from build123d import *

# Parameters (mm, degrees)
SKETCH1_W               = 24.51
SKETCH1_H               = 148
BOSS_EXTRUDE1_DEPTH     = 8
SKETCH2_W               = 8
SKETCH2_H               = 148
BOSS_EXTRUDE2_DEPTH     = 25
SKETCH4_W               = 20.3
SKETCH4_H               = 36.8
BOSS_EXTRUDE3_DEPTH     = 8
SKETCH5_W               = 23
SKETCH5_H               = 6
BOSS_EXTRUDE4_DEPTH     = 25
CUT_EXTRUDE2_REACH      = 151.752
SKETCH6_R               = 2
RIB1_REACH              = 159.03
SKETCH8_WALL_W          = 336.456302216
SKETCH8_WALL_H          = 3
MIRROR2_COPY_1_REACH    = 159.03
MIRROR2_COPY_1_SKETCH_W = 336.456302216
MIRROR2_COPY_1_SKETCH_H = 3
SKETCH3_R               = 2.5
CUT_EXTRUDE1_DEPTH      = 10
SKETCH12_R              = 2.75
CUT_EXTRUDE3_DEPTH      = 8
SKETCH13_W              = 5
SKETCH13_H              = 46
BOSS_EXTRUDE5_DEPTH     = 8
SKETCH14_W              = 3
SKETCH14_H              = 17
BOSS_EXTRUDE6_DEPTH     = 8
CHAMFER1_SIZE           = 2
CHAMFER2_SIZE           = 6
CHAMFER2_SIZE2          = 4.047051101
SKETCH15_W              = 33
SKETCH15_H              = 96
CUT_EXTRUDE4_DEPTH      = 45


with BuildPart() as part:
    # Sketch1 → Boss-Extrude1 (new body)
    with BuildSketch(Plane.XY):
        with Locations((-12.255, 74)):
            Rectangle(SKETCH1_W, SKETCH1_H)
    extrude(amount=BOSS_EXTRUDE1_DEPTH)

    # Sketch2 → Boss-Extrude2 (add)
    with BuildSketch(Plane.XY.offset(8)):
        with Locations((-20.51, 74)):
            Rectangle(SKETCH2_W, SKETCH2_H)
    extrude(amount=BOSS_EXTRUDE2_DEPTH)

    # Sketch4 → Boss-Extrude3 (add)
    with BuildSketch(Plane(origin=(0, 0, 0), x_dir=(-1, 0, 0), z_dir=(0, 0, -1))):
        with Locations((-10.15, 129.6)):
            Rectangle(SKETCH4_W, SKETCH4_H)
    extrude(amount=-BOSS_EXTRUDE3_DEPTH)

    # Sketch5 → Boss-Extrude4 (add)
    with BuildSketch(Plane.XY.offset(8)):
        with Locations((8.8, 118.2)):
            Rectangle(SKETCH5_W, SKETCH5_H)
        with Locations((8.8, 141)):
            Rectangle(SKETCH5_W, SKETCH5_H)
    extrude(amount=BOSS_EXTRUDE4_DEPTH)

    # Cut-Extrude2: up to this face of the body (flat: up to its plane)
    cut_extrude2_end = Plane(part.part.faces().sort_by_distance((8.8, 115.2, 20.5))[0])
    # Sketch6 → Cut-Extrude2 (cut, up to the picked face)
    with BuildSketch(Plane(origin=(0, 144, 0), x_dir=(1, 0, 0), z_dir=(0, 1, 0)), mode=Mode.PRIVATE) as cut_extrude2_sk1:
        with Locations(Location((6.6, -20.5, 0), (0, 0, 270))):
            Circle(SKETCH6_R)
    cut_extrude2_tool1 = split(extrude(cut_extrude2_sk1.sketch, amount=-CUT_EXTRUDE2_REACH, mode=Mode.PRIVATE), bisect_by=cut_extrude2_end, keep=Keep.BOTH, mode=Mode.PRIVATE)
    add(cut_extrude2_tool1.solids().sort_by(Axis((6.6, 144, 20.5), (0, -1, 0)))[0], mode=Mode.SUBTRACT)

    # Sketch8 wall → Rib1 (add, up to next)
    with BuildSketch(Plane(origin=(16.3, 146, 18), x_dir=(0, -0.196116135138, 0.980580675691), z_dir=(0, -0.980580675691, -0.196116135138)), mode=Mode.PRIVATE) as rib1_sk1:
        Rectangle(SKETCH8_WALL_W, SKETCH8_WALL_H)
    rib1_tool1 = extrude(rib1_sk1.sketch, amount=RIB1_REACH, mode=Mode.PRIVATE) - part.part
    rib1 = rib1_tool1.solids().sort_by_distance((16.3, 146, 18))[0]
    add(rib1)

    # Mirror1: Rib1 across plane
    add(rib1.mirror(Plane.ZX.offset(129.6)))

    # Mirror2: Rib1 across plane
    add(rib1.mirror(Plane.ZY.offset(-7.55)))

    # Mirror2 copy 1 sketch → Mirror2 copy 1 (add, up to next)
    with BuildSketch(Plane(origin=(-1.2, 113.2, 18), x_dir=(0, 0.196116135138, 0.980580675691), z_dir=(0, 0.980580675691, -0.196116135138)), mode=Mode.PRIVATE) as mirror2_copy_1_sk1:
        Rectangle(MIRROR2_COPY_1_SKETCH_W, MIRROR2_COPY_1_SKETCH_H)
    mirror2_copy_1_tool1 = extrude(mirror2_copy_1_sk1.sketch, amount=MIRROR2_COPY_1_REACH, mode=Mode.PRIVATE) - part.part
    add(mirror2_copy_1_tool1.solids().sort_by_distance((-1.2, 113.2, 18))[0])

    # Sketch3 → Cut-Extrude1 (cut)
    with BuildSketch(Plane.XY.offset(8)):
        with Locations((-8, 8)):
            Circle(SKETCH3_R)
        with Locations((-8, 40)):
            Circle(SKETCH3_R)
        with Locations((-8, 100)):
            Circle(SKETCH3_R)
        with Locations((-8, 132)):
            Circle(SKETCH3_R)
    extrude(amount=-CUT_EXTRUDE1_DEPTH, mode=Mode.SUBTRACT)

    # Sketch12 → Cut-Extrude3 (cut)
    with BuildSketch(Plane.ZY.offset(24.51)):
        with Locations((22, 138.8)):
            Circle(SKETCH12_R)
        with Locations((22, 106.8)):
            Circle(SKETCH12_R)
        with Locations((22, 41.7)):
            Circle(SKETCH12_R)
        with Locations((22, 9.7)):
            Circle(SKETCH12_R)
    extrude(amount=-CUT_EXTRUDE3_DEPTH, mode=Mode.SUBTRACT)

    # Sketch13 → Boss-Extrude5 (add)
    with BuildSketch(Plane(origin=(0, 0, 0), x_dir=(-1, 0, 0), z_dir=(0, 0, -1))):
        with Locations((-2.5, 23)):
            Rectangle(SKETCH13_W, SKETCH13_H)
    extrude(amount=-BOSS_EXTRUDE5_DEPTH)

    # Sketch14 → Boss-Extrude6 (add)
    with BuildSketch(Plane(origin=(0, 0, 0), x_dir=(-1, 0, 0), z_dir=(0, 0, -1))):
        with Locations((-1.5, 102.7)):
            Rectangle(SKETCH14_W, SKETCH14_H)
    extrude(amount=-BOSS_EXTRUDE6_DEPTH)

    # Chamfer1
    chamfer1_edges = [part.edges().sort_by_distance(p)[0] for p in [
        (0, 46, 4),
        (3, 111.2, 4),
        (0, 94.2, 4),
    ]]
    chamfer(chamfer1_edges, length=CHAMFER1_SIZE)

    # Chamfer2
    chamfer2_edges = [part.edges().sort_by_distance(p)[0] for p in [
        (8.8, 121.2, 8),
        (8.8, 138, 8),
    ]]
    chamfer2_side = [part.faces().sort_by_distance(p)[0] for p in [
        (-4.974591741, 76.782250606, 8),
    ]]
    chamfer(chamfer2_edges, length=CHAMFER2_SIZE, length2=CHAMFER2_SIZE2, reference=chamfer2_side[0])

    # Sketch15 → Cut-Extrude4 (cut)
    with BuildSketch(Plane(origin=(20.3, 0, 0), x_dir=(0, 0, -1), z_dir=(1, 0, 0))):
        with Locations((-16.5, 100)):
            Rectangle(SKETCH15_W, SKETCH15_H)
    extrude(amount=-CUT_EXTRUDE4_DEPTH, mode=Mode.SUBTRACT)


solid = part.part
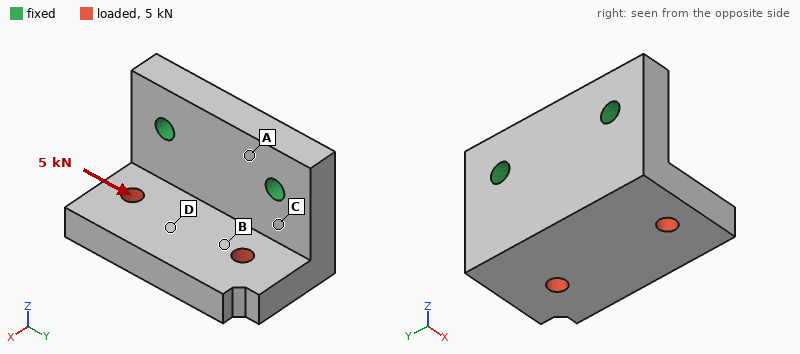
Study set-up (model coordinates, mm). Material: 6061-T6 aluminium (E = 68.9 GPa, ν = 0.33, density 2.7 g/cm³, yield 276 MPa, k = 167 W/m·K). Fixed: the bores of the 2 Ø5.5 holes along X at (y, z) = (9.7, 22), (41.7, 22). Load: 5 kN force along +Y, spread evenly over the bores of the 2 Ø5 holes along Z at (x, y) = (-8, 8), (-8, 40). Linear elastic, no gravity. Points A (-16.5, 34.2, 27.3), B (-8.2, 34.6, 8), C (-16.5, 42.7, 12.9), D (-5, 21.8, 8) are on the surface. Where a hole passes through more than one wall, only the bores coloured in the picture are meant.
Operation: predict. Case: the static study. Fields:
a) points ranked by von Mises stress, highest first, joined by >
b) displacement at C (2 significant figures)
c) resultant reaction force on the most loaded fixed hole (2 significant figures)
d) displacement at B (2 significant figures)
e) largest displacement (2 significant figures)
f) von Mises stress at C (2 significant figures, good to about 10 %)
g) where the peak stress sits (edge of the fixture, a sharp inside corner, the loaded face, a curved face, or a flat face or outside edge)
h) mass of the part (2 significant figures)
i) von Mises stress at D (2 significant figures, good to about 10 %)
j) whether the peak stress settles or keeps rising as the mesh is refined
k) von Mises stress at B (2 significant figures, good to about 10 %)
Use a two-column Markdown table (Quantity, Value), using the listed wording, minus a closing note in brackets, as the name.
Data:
| Quantity | Value |
|---|---|
| points ranked by von Mises stress, highest first, joined by > | C > B > D > A |
| displacement at C | 15 µm |
| resultant reaction force on the most loaded fixed hole | 3.9 kN |
| displacement at B | 38 µm |
| largest displacement | 72 µm |
| von Mises stress at C | 52 MPa |
| where the peak stress sits | edge of the fixture |
| mass of the part | 59 g |
| von Mises stress at D | 22 MPa |
| whether the peak stress settles or keeps rising as the mesh is refined | keeps rising |
| von Mises stress at B | 39 MPa |
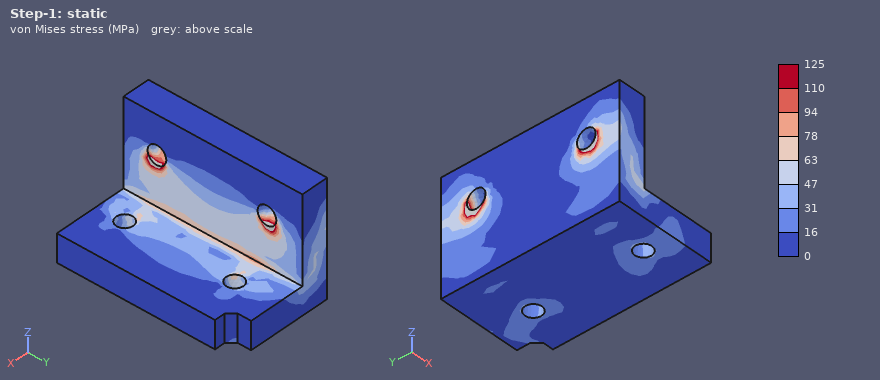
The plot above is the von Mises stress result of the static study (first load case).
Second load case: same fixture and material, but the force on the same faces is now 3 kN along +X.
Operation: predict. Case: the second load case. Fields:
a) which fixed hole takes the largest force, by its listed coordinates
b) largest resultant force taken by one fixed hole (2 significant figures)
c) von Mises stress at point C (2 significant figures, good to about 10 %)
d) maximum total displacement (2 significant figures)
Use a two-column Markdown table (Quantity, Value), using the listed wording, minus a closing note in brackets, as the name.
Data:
| Quantity | Value |
|---|---|
| which fixed hole takes the largest force, by its listed coordinates | (9.7, 22) |
| largest resultant force taken by one fixed hole | 1.6 kN |
| von Mises stress at point C | 51 MPa |
| maximum total displacement | 0.11 mm |
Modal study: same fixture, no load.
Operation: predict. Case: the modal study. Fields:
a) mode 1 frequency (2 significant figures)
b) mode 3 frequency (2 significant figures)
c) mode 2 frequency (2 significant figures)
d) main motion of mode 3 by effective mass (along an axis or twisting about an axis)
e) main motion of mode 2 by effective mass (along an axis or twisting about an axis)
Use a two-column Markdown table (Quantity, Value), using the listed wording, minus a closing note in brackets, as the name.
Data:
| Quantity | Value |
|---|---|
| mode 1 frequency | 4600 Hz |
| mode 3 frequency | 12 kHz |
| mode 2 frequency | 7800 Hz |
| main motion of mode 3 by effective mass | along X |
| main motion of mode 2 by effective mass | along Y |
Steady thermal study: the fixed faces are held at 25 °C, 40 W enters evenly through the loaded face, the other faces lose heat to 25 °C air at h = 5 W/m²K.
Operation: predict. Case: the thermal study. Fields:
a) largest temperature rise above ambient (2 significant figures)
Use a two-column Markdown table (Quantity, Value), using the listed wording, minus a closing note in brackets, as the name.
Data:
| Quantity | Value |
|---|---|
| largest temperature rise above ambient | 20 K |
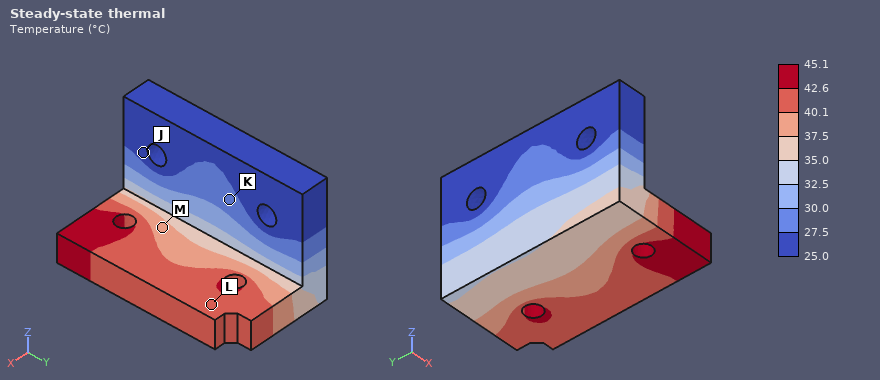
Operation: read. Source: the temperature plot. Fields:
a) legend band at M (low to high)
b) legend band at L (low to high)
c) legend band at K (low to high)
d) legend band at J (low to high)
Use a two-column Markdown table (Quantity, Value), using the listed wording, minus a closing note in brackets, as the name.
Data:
| Quantity | Value |
|---|---|
| legend band at M | 37.5 to 40.1 °C |
| legend band at L | 40.1 to 42.6 °C |
| legend band at K | 27.5 to 30.0 °C |
| legend band at J | 25.0 to 27.5 °C |
